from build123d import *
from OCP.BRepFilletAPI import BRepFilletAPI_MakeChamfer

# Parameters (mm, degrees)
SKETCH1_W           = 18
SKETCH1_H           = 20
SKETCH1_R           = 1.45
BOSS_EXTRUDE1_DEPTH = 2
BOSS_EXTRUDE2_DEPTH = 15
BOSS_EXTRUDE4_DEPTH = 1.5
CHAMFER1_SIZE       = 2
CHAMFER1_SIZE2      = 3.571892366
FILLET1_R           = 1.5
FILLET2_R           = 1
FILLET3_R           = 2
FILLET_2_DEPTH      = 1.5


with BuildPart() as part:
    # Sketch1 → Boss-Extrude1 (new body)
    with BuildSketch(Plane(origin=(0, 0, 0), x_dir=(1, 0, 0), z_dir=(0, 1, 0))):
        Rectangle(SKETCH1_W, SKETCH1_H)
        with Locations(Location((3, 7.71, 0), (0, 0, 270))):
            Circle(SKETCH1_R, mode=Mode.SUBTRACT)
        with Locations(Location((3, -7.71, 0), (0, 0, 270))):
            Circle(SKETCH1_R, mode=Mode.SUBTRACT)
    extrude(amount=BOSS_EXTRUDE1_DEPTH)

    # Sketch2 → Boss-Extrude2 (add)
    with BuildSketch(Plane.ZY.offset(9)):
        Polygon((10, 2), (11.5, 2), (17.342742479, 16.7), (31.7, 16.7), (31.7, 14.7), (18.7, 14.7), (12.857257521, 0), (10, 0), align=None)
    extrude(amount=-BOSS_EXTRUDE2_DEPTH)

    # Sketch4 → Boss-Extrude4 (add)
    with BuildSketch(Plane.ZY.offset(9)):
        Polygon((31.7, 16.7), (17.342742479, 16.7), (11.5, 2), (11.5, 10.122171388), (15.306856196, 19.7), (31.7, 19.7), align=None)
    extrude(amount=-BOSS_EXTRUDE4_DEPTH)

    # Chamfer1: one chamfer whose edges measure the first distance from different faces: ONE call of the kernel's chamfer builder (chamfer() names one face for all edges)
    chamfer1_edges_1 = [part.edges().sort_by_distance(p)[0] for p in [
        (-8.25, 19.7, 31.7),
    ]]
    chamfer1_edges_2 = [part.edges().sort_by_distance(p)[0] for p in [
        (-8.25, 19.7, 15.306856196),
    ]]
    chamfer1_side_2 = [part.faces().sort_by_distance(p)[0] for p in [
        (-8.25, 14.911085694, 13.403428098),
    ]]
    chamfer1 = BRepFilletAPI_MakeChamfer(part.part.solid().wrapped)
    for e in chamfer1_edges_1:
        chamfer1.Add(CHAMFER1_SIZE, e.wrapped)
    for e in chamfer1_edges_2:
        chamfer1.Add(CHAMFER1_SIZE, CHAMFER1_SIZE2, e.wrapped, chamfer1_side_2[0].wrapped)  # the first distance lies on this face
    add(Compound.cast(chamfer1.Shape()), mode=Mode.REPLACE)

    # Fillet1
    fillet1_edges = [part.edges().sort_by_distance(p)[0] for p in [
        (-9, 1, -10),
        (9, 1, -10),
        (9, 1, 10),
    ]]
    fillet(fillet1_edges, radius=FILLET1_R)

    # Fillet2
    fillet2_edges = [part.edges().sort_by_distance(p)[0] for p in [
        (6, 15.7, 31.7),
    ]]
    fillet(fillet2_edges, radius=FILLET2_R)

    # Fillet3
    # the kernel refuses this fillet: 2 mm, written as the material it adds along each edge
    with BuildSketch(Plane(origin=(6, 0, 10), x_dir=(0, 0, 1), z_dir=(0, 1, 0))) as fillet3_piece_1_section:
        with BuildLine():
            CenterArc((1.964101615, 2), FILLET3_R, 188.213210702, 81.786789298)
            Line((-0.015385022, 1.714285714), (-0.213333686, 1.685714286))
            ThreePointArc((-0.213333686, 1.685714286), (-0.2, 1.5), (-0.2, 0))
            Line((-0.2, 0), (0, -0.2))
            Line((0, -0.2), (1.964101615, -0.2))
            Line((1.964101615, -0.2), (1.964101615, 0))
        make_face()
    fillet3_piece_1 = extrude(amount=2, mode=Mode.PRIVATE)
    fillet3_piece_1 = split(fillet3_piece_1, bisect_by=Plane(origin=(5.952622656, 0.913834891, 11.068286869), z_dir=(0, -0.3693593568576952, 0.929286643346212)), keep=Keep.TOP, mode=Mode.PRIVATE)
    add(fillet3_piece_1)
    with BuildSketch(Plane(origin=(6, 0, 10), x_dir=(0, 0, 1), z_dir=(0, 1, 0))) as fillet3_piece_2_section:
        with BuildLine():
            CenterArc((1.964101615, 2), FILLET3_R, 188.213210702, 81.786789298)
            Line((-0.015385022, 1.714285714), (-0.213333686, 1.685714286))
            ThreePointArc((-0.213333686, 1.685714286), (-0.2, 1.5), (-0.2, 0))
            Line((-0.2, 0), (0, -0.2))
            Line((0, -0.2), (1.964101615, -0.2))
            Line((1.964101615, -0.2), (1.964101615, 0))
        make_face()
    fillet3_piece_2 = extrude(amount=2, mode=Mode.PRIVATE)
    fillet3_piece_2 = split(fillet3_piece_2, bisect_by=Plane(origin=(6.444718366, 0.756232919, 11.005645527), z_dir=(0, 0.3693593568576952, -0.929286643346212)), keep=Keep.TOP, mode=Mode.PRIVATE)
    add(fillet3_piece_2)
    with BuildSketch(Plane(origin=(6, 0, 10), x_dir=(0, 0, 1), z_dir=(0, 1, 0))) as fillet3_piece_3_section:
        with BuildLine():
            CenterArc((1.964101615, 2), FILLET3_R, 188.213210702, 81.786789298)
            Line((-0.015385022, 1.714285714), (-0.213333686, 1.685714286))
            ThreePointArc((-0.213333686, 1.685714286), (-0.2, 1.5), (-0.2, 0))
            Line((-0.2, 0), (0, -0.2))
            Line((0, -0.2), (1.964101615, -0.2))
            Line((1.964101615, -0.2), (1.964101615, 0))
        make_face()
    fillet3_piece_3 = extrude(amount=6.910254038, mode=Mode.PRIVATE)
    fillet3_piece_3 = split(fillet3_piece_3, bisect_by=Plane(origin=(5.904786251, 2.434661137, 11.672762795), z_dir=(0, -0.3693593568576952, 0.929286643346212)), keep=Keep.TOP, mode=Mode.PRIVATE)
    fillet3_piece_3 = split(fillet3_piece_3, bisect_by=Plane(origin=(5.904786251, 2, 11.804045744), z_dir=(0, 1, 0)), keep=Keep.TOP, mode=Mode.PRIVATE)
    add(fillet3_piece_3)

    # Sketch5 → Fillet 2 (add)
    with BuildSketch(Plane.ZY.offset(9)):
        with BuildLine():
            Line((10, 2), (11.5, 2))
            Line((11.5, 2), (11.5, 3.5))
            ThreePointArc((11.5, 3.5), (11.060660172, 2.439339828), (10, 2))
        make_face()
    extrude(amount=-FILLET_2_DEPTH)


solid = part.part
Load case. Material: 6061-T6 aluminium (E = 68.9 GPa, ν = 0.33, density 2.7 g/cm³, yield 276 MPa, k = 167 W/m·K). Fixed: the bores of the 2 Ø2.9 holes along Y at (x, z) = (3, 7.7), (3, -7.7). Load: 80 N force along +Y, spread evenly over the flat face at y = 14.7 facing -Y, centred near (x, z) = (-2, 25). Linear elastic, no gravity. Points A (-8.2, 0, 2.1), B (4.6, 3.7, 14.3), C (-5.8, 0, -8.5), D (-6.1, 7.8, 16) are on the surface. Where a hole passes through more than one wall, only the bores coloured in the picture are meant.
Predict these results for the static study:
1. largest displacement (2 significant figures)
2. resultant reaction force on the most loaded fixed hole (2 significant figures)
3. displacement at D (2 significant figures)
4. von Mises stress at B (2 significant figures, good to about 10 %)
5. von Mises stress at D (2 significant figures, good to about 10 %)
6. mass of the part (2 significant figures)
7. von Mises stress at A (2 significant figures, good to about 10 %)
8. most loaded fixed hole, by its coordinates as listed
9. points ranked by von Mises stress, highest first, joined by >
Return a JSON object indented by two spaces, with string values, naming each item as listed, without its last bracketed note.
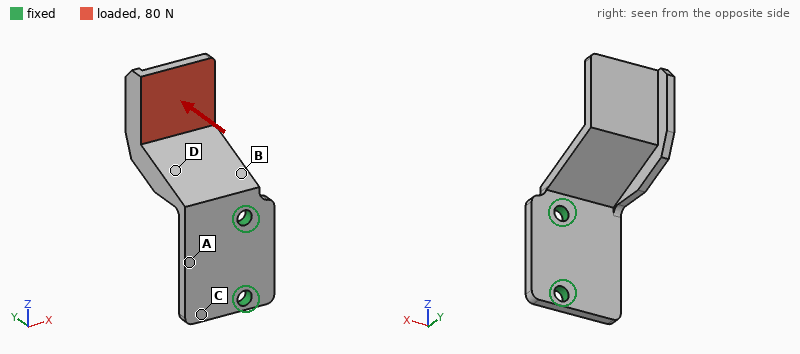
{
  "largest displacement": "0.50 mm",
  "resultant reaction force on the most loaded fixed hole": "110 N",
  "displacement at D": "0.13 mm",
  "von Mises stress at B": "91 MPa",
  "von Mises stress at D": "48 MPa",
  "mass of the part": "4.8 g",
  "von Mises stress at A": "33 MPa",
  "most loaded fixed hole, by its coordinates as listed": "(3, 7.7)",
  "points ranked by von Mises stress, highest first, joined by >": "B > D > A > C"
}
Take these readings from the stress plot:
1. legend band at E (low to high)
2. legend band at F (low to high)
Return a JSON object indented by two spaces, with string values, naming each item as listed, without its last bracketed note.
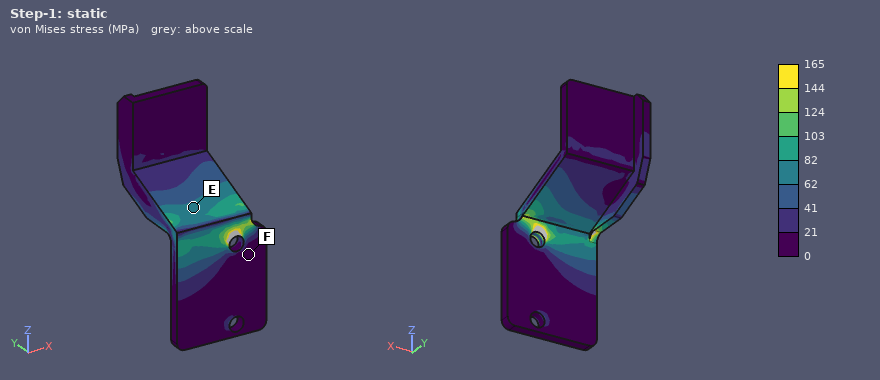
{
  "legend band at E": "62 to 82 MPa",
  "legend band at F": "0 to 21 MPa"
}
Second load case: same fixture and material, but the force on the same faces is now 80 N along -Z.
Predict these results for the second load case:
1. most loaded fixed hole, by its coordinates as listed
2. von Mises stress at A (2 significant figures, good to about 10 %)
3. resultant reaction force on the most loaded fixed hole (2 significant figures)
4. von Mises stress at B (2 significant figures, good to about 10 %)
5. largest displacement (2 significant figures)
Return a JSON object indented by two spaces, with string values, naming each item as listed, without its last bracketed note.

{
  "most loaded fixed hole, by its coordinates as listed": "(3, 7.7)",
  "von Mises stress at A": "24 MPa",
  "resultant reaction force on the most loaded fixed hole": "69 N",
  "von Mises stress at B": "83 MPa",
  "largest displacement": "0.38 mm"
}
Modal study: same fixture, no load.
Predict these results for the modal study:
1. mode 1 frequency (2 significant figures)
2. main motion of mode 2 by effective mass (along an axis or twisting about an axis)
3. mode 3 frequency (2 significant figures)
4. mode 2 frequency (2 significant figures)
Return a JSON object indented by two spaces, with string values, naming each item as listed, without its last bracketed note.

{
  "mode 1 frequency": "1600 Hz",
  "main motion of mode 2 by effective mass": "along X",
  "mode 3 frequency": "5200 Hz",
  "mode 2 frequency": "3500 Hz"
}
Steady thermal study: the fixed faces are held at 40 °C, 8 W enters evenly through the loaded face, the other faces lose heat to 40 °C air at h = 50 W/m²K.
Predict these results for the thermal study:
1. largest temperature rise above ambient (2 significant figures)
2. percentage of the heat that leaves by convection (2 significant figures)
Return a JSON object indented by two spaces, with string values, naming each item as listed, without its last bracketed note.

{
  "largest temperature rise above ambient": "38 K",
  "percentage of the heat that leaves by convection": "16 %"
}
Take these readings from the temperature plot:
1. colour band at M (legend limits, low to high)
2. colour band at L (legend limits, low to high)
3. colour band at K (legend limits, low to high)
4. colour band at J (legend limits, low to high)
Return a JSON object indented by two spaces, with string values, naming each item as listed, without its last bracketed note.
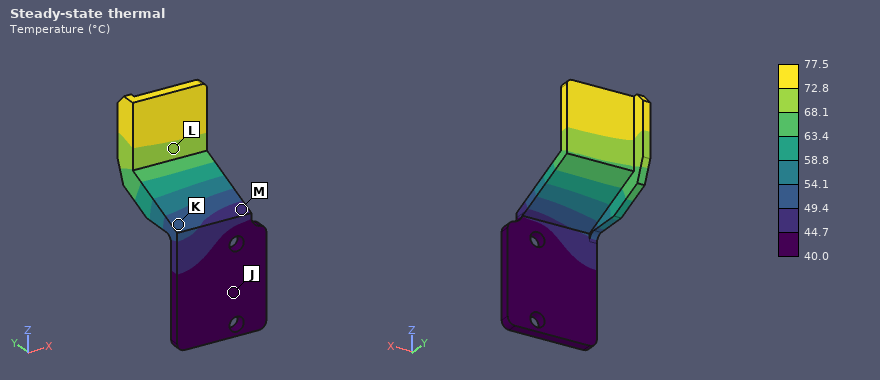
{
  "colour band at M": "44.7 to 49.4 °C",
  "colour band at L": "68.1 to 72.8 °C",
  "colour band at K": "49.4 to 54.1 °C",
  "colour band at J": "40.0 to 44.7 °C"
}
